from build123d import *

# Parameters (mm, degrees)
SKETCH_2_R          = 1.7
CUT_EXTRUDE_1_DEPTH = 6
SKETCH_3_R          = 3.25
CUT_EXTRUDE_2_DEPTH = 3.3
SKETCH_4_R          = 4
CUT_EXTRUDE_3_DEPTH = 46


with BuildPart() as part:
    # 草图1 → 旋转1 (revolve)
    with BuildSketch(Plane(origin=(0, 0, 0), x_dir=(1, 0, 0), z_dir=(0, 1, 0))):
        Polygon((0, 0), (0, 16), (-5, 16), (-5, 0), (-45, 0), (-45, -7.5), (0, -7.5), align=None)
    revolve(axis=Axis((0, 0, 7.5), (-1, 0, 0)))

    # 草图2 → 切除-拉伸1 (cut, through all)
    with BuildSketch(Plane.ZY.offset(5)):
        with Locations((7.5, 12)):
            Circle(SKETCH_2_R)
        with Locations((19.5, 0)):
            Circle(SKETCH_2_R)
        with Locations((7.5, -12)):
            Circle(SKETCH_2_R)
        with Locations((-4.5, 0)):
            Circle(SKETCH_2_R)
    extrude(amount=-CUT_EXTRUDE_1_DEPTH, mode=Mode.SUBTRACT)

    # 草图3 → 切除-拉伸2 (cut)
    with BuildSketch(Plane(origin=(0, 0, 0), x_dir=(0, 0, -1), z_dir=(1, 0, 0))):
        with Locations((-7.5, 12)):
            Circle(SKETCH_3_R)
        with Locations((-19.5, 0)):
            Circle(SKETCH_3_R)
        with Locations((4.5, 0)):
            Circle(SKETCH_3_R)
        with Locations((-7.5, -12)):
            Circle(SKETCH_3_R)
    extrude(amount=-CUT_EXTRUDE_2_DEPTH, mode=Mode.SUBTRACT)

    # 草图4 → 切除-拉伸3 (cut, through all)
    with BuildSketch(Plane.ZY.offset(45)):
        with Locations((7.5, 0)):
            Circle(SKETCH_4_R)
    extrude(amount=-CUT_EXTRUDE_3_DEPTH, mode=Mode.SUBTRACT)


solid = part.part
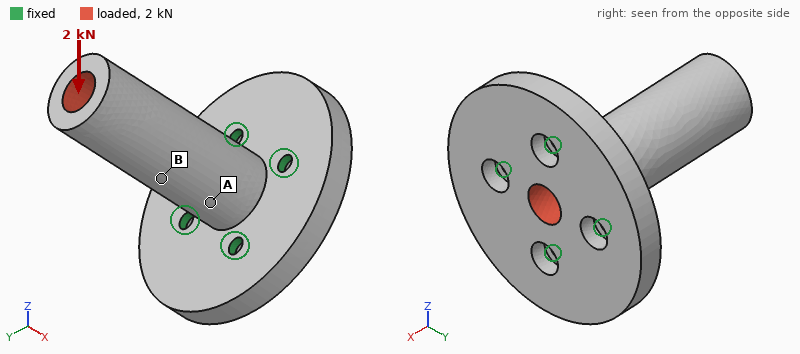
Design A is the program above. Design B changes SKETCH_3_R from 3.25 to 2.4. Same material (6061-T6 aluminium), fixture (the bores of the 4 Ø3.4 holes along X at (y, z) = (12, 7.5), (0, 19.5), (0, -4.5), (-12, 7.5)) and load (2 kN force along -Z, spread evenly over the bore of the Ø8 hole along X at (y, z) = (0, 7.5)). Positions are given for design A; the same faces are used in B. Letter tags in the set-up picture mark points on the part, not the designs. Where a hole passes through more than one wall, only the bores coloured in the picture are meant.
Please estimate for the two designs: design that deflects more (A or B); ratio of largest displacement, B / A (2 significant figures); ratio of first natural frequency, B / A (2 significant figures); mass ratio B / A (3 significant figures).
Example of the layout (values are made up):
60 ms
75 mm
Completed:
A
0.92
1.0
1.02
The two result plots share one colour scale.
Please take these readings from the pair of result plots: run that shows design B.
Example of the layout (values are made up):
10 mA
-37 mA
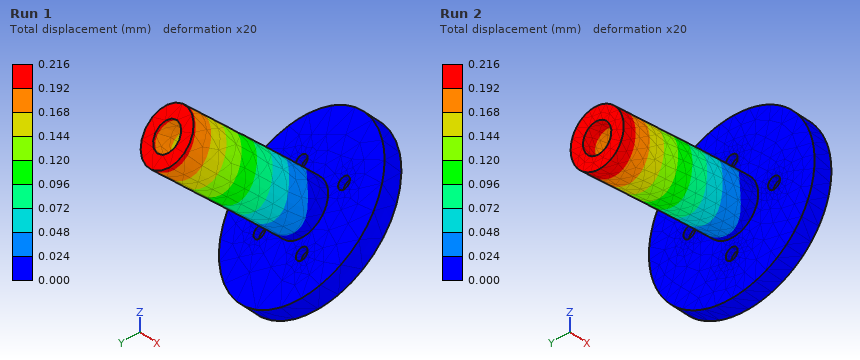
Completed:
Run 1
